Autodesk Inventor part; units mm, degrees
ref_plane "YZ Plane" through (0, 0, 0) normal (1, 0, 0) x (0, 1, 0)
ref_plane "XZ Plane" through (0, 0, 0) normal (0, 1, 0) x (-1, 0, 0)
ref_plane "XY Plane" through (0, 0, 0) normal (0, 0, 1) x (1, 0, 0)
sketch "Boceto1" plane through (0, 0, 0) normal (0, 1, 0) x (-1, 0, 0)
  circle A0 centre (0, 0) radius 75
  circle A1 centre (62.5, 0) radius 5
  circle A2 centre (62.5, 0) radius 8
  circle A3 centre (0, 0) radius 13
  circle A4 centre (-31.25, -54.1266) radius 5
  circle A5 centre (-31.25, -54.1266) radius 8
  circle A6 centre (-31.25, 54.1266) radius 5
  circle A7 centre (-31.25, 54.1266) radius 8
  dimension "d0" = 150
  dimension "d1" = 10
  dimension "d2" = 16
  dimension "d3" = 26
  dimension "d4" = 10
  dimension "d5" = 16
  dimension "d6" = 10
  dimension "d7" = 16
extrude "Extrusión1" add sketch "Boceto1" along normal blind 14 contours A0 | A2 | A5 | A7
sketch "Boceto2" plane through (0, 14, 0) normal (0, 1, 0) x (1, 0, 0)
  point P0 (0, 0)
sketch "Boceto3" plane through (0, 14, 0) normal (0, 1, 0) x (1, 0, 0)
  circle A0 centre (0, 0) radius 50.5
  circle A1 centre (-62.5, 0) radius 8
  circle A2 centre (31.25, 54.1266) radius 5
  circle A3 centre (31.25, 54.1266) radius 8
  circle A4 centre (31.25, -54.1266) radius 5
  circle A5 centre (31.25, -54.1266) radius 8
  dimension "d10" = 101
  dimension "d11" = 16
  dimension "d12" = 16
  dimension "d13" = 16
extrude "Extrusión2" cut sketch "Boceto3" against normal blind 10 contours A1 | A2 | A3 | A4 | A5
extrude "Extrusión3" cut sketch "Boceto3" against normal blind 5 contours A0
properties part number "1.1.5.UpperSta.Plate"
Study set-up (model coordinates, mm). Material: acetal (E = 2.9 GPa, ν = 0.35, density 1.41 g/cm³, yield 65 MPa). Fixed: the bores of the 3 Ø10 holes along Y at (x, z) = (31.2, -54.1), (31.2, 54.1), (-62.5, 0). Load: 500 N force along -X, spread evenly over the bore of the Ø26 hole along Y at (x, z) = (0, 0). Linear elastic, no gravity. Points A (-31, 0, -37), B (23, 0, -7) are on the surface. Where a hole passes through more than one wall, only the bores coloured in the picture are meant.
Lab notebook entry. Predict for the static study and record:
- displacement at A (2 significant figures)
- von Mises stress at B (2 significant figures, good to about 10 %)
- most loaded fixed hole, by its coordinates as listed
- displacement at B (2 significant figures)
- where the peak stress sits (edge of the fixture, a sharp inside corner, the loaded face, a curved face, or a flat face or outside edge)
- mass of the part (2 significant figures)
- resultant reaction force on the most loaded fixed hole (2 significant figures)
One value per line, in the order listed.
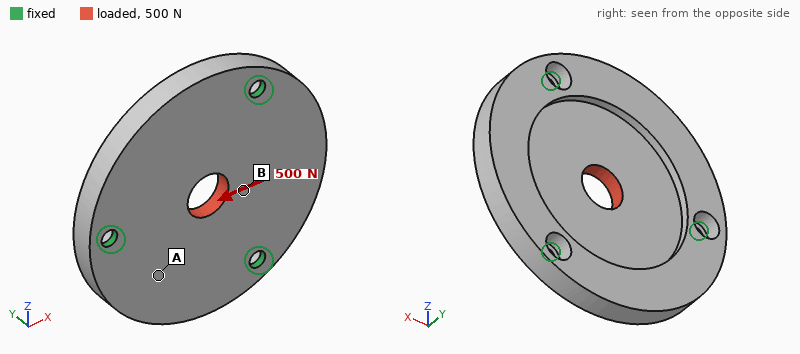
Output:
9.5 µm
0.56 MPa
(-62.5, 0)
14 µm
edge of the fixture
280 g
180 N
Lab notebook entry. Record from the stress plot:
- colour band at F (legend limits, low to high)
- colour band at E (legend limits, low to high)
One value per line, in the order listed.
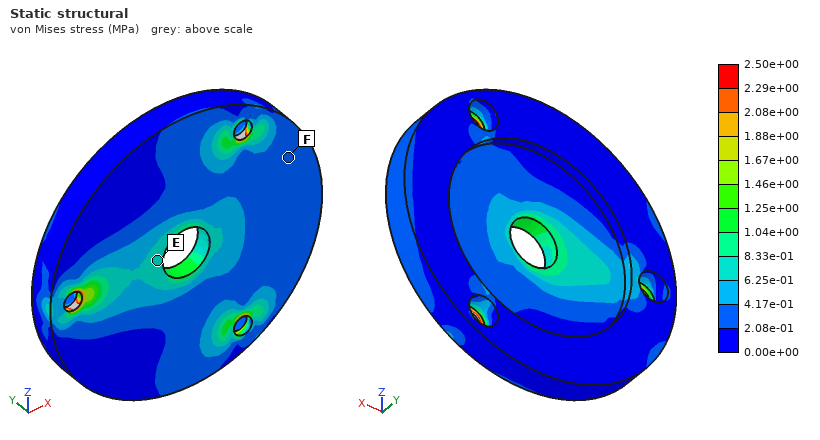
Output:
2.08e-01 to 4.17e-01 MPa
6.25e-01 to 8.33e-01 MPa
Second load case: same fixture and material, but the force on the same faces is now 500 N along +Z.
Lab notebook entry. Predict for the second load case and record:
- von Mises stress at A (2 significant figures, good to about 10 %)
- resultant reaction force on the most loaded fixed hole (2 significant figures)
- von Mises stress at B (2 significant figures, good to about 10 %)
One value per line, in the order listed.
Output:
0.26 MPa
170 N
0.45 MPa
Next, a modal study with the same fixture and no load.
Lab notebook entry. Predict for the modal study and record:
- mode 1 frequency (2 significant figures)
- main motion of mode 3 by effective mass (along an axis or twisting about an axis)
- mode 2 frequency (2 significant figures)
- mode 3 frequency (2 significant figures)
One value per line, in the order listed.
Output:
650 Hz
along Y
650 Hz
900 Hz
